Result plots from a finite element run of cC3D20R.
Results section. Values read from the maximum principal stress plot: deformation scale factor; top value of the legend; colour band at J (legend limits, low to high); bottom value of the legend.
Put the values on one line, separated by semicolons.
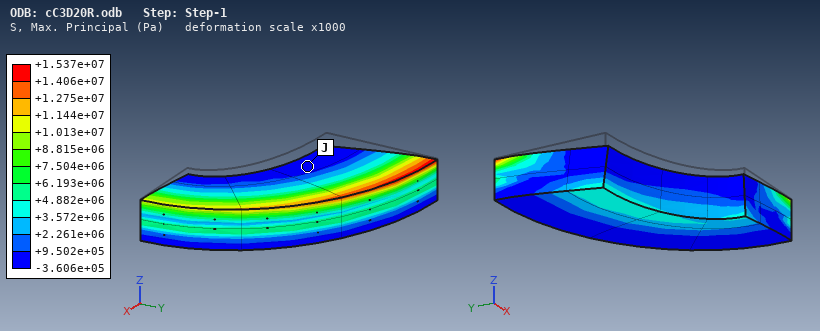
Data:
1000; +1.537e+07 Pa; -3.606e+05 to +9.502e+05 Pa; -3.606e+05 Pa
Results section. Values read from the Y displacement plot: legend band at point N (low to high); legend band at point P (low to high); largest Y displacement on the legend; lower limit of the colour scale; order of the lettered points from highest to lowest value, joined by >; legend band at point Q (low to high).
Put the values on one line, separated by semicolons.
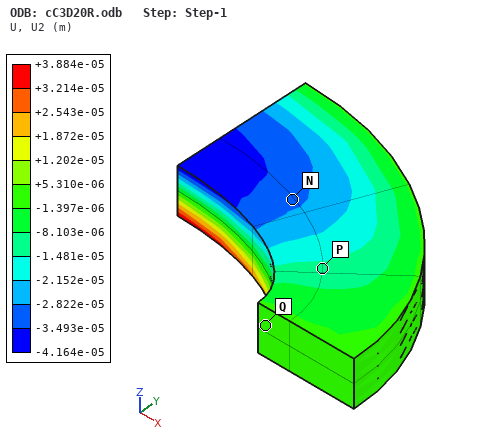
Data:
-3.493e-05 to -2.822e-05 m; -1.481e-05 to -8.103e-06 m; +3.884e-05 m; -4.164e-05 m; Q > P > N; -1.397e-06 to +5.310e-06 m
